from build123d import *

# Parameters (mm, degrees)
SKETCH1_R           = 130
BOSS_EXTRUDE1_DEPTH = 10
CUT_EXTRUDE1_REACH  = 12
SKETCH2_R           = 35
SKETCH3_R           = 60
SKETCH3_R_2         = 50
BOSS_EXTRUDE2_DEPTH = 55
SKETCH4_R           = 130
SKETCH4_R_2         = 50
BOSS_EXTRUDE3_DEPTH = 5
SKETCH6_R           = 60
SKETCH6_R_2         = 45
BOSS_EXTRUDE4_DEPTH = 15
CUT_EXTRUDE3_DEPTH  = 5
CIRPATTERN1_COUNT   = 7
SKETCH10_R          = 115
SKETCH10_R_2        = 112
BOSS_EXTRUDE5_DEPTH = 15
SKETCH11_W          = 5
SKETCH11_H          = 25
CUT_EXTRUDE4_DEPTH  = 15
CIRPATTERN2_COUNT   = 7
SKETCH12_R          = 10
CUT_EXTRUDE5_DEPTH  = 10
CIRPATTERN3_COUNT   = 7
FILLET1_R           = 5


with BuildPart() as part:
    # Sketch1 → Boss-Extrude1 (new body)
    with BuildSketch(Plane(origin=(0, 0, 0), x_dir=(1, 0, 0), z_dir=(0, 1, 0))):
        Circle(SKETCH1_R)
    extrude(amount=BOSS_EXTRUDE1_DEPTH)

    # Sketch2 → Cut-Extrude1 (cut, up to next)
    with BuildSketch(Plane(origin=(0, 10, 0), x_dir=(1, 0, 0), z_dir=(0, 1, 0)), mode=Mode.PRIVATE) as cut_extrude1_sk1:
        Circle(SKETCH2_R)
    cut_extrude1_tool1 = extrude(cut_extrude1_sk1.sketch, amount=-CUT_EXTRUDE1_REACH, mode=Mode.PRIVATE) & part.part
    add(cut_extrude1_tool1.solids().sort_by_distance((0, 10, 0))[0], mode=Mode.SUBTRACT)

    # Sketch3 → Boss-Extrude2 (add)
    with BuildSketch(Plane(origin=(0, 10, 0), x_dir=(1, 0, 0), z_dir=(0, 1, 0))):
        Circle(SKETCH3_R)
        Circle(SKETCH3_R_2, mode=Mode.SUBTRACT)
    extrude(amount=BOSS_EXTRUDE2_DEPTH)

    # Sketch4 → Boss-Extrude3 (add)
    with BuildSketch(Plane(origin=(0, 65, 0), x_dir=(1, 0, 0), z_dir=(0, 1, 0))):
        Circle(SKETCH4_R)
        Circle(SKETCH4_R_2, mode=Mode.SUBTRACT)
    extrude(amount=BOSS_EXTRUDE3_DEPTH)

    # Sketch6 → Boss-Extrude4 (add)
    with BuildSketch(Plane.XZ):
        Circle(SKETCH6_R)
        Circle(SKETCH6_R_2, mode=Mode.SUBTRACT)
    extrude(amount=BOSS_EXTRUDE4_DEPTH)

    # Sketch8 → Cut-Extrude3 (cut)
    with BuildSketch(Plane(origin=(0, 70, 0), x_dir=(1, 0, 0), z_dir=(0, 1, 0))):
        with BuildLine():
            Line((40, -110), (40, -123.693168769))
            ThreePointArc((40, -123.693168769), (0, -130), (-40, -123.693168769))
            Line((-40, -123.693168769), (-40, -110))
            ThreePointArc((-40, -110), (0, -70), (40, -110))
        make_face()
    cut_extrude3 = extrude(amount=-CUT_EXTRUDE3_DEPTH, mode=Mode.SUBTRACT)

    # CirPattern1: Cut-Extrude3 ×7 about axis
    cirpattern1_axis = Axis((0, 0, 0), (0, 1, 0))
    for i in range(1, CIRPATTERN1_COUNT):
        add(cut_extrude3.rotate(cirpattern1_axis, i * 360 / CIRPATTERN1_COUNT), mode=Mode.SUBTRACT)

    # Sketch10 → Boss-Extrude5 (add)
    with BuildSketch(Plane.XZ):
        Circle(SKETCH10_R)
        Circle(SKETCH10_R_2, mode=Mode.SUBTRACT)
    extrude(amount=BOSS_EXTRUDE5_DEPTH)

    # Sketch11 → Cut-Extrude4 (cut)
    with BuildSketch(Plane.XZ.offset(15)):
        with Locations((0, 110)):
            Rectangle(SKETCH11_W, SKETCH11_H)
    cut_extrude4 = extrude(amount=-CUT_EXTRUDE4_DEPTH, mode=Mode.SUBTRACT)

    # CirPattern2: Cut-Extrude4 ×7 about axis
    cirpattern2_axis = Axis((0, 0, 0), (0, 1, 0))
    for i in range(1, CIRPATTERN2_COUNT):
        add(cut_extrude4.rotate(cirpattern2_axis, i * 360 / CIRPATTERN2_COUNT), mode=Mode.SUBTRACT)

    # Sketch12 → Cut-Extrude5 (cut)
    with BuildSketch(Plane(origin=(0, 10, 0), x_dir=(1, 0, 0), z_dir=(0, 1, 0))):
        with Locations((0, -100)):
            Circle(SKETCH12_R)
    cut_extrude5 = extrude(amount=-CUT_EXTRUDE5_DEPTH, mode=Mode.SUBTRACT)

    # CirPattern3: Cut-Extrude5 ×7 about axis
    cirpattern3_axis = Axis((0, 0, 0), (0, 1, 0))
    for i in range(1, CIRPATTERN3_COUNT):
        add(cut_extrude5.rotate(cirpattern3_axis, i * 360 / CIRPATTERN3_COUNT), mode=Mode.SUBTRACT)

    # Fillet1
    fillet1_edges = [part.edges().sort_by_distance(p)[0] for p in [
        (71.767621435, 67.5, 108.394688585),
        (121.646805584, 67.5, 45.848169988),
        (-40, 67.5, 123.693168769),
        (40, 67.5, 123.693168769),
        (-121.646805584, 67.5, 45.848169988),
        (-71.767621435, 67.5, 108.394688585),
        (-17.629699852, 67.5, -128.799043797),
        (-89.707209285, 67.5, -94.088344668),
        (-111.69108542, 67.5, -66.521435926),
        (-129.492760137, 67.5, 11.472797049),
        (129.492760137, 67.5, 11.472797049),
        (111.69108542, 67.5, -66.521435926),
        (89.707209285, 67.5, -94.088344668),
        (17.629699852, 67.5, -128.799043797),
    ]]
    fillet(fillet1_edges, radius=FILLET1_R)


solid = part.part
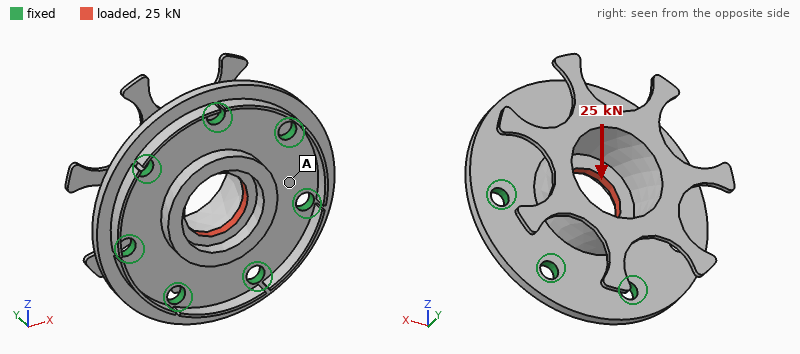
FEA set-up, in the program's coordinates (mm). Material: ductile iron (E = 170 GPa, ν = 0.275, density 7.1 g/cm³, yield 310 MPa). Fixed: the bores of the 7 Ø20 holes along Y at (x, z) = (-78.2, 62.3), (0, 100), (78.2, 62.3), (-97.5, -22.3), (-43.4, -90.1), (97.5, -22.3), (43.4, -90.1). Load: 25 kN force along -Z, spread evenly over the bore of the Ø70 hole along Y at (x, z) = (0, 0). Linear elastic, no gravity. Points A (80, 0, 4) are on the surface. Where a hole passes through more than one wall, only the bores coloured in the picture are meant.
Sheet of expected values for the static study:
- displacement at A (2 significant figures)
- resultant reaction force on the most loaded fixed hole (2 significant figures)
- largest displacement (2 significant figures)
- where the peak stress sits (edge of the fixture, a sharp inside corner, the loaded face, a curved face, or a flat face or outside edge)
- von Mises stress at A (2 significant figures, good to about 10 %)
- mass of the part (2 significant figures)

0.64 µm
5.4 kN
4.0 µm
a sharp inside corner
3.6 MPa
6.1 kg
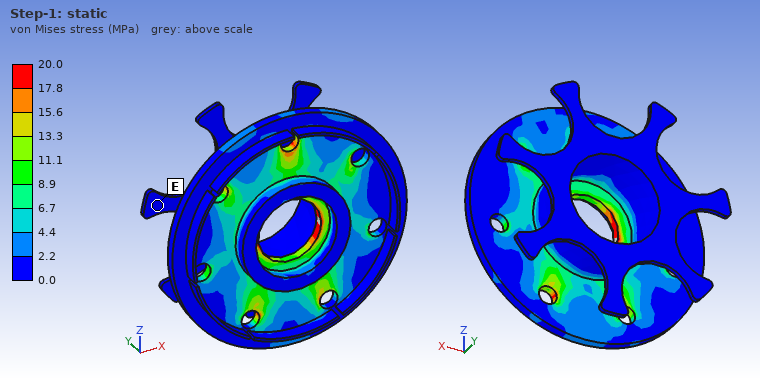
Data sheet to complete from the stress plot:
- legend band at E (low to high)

0.0 to 2.2 MPa
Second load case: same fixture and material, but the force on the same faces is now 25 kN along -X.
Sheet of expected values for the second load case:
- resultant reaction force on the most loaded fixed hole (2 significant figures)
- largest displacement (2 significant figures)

5.3 kN
4.0 µm
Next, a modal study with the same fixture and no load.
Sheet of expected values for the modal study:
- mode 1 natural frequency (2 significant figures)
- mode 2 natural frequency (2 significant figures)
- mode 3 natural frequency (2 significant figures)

850 Hz
860 Hz
870 Hz
